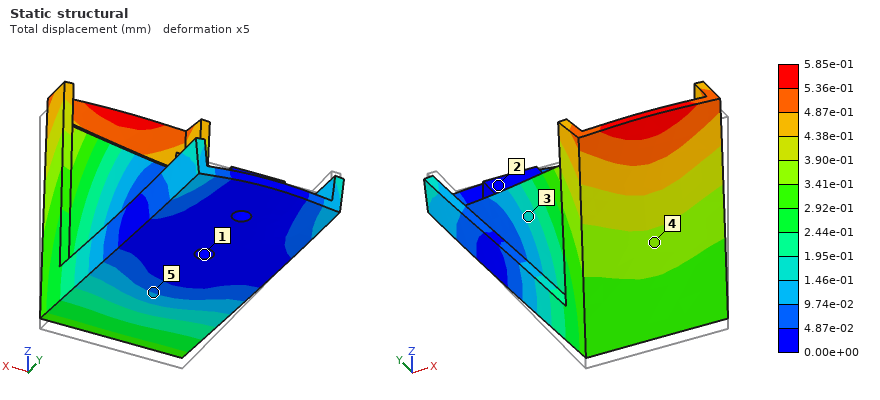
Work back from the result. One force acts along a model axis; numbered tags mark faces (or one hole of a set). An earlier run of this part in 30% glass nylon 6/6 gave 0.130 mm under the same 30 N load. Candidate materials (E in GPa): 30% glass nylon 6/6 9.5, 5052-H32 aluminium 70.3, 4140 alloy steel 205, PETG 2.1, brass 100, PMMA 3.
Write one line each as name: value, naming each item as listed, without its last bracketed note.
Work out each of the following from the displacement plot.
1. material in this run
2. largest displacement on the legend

material in this run: PETG
largest displacement on the legend: 5.85e-01 mm
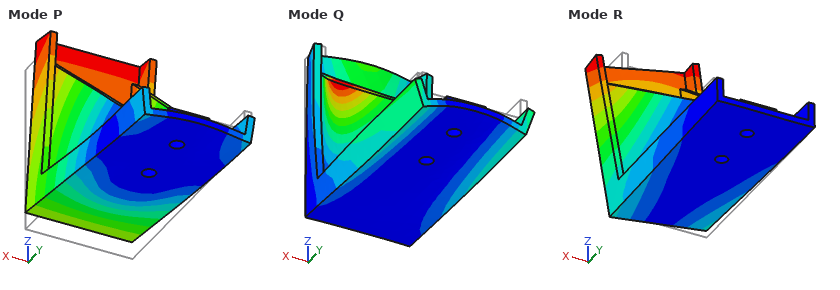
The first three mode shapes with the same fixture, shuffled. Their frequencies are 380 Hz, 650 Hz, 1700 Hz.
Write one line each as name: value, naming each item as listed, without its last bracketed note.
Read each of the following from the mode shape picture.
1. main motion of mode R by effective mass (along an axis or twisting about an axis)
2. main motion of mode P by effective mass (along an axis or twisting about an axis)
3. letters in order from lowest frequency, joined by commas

main motion of mode R by effective mass: along X
main motion of mode P by effective mass: along Z
letters in order from lowest frequency, joined by commas: R, P, Q
